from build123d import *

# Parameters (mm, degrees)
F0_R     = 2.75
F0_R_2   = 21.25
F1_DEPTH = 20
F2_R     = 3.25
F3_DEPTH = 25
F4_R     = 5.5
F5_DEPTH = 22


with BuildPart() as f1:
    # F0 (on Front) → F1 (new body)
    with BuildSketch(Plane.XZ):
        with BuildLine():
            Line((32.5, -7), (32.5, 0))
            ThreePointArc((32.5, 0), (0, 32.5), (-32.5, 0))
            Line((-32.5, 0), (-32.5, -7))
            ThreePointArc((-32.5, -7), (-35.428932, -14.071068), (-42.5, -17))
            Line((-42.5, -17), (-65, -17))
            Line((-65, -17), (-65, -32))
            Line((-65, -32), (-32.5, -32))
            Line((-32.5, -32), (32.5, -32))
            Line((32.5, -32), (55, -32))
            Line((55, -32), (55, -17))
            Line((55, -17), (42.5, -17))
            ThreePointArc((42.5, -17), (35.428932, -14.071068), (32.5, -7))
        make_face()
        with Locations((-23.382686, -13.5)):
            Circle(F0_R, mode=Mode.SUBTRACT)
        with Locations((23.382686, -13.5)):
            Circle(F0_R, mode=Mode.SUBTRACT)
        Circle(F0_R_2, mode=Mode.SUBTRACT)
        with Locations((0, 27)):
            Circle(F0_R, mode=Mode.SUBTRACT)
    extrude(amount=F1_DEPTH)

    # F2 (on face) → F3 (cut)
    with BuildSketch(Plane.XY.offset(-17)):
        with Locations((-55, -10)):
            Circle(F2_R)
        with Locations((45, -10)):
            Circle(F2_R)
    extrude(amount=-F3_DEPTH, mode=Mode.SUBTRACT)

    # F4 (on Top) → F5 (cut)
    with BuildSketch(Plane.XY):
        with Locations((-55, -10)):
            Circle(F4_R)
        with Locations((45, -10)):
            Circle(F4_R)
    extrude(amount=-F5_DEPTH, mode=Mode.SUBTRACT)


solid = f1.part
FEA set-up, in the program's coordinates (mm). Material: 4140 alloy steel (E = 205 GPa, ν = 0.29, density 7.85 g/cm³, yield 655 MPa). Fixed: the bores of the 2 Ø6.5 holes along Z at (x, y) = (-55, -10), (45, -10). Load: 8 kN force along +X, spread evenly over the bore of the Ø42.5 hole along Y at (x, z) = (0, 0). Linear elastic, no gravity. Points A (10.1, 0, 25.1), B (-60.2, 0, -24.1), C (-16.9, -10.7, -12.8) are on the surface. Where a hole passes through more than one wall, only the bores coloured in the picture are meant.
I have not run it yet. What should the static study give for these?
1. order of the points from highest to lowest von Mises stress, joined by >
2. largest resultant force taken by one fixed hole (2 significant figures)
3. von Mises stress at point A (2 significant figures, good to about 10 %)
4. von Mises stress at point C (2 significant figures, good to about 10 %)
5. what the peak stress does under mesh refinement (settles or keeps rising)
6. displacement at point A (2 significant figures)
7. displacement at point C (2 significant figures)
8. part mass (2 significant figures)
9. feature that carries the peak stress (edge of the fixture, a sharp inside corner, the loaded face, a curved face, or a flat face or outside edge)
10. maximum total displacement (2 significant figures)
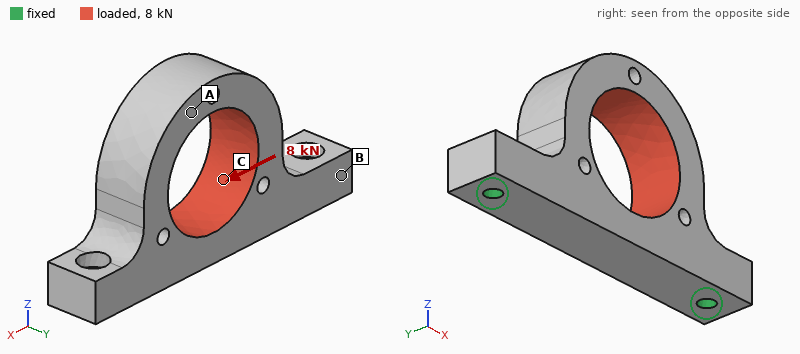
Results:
C > A > B
4.6 kN
12 MPa
44 MPa
keeps rising
22 µm
3.5 µm
480 g
edge of the fixture
23 µm
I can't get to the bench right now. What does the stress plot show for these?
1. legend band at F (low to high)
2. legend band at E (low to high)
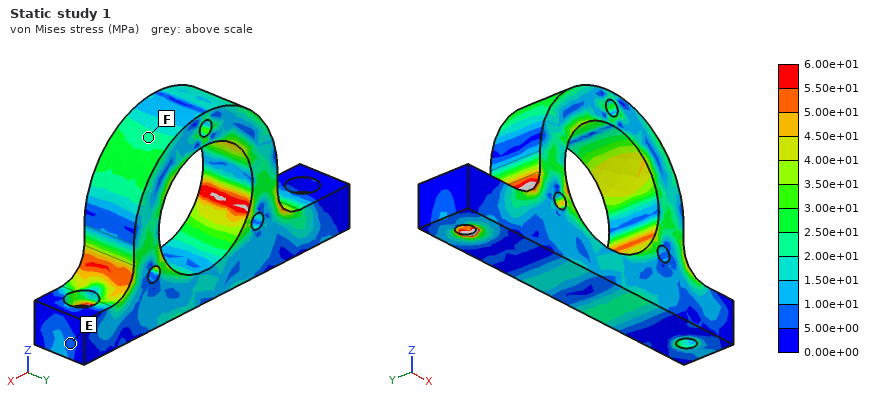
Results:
2.00e+01 to 2.50e+01 MPa
5.00e+00 to 1.00e+01 MPa
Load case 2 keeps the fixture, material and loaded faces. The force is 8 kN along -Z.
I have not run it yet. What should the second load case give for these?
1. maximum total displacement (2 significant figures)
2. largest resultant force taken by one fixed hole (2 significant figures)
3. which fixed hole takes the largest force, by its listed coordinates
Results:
23 µm
4.7 kN
(45, -10)
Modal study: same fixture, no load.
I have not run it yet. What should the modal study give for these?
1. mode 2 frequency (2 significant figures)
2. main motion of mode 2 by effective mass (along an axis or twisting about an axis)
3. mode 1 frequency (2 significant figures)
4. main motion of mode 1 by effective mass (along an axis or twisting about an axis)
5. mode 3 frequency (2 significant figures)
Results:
5500 Hz
along Z
2300 Hz
along Y
6300 Hz
